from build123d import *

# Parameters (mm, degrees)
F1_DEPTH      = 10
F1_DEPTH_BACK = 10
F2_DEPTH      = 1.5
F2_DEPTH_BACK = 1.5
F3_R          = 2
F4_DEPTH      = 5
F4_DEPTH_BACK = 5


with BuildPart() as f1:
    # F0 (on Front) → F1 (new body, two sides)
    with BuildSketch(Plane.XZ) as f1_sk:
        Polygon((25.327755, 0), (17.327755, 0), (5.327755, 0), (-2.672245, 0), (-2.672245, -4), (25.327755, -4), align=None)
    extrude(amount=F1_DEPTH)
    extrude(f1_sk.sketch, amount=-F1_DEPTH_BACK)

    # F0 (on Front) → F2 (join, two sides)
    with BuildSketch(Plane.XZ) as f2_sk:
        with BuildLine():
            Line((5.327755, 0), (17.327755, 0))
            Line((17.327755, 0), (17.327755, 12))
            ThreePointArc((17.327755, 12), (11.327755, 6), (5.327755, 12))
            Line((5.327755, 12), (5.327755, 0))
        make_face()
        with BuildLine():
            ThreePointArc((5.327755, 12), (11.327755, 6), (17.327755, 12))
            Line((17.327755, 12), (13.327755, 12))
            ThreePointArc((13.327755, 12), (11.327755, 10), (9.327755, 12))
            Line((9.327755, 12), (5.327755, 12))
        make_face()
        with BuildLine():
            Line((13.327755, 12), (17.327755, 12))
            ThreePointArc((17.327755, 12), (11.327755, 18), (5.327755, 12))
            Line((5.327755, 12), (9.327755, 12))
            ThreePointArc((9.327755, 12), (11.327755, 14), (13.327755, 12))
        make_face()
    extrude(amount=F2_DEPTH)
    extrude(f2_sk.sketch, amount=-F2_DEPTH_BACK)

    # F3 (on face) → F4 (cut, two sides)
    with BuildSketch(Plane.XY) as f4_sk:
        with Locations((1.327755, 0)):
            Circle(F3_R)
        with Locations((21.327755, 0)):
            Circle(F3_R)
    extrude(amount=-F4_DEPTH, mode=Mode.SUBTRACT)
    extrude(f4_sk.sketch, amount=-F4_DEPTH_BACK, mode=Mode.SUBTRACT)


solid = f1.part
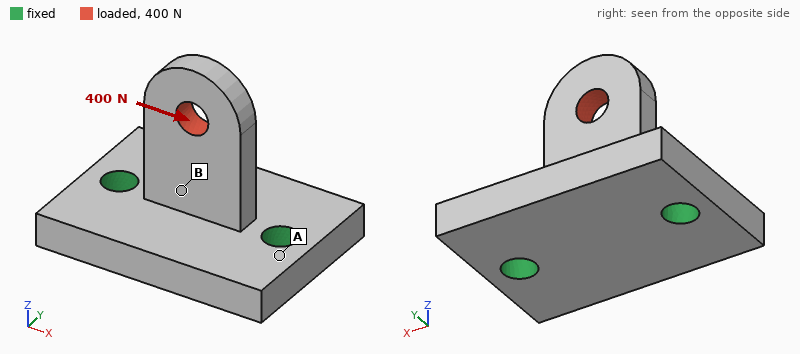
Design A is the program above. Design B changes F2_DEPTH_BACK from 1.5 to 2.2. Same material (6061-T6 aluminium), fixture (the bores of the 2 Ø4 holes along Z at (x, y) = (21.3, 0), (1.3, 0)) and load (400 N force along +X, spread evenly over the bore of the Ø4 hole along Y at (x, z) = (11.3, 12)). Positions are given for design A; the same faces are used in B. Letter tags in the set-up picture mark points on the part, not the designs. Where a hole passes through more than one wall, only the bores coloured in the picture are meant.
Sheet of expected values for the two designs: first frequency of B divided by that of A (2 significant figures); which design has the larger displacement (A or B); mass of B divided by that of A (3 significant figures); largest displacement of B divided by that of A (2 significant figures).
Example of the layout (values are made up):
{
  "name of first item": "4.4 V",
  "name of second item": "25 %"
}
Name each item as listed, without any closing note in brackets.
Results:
{
  "first frequency of B divided by that of A": "1.1",
  "which design has the larger displacement": "A",
  "mass of B divided by that of A": "1.05",
  "largest displacement of B divided by that of A": "0.84"
}
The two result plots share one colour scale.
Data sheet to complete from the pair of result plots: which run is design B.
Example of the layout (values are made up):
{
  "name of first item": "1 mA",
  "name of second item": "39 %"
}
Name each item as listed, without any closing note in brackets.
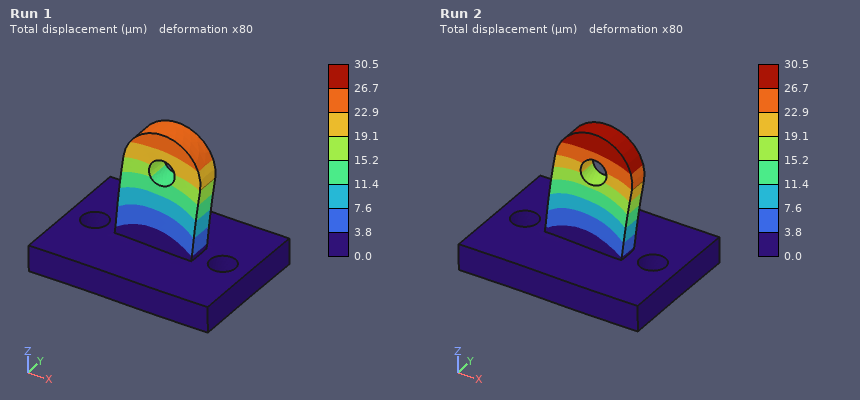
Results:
{
  "which run is design B": "Run 1"
}
